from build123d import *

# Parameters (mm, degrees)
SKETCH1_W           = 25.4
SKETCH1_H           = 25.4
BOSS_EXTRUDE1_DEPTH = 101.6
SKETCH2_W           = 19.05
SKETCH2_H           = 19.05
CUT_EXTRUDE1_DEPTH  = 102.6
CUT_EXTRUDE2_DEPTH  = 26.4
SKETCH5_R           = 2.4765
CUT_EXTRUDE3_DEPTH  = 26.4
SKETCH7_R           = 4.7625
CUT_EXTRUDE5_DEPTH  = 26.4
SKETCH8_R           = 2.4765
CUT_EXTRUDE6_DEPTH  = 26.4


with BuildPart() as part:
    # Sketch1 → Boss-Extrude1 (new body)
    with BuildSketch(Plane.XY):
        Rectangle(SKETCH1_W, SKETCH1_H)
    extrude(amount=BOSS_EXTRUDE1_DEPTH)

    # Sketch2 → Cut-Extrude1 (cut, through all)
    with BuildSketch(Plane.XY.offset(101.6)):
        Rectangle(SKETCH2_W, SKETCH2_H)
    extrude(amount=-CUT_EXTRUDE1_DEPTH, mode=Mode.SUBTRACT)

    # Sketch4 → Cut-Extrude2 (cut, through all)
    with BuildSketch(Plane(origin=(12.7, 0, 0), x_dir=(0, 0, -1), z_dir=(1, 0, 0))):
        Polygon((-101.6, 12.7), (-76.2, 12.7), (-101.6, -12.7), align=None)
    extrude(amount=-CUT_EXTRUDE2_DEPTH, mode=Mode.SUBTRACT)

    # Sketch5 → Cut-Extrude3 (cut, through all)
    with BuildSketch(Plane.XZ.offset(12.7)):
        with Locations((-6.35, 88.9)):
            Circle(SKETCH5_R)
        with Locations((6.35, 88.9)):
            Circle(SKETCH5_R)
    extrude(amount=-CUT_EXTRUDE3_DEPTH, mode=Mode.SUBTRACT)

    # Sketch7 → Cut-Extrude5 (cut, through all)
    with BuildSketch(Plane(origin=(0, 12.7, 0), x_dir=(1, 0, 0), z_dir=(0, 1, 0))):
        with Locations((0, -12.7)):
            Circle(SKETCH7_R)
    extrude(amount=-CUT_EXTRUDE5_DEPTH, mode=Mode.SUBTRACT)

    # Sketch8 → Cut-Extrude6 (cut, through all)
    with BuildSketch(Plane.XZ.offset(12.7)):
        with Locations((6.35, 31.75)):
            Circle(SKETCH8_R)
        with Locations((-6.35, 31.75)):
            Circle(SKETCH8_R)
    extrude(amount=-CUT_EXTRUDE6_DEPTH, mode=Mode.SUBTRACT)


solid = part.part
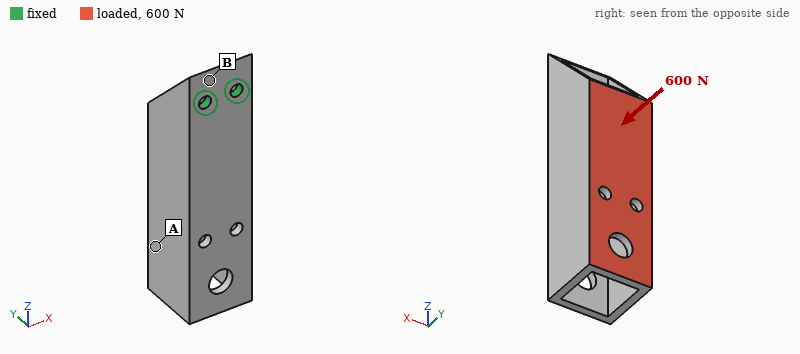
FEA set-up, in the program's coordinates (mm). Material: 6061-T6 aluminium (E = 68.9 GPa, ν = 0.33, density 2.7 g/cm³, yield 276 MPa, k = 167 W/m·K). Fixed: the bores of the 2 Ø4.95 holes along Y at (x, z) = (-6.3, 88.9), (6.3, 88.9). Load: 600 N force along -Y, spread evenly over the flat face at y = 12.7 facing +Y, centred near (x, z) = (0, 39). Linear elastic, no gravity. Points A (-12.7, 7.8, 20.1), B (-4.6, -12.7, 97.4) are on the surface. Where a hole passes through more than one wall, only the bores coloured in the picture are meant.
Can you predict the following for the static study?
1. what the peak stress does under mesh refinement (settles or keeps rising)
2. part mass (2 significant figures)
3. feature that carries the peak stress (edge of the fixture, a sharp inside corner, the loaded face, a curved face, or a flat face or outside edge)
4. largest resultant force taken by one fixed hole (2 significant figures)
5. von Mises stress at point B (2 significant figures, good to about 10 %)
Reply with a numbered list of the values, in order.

1. keeps rising
2. 66 g
3. edge of the fixture
4. 310 N
5. 72 MPa
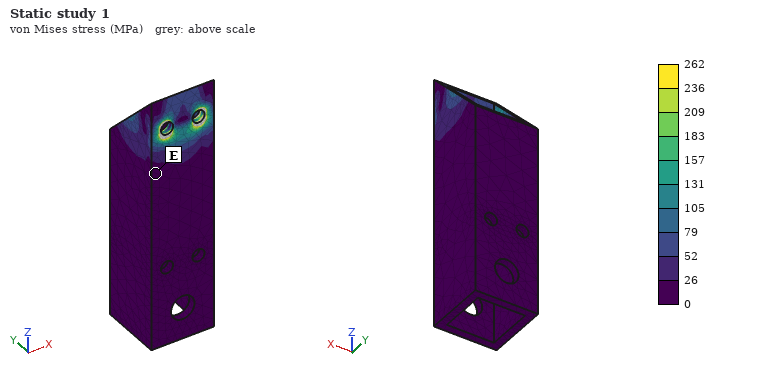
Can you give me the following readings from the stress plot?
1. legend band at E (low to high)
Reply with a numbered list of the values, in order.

1. 0 to 26 MPa
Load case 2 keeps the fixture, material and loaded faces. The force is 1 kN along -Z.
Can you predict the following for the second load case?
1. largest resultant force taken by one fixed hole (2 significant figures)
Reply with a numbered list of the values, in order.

1. 500 N
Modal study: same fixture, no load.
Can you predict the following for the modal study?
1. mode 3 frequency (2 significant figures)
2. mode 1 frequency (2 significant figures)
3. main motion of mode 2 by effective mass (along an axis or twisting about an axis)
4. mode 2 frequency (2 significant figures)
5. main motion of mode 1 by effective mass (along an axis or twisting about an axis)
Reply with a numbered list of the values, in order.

1. 2700 Hz
2. 690 Hz
3. along X
4. 1700 Hz
5. along Y
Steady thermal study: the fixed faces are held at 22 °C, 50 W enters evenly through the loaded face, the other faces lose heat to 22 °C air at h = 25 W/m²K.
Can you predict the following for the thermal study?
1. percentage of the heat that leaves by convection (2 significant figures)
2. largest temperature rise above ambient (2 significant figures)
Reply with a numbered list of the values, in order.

1. 29 %
2. 60 K
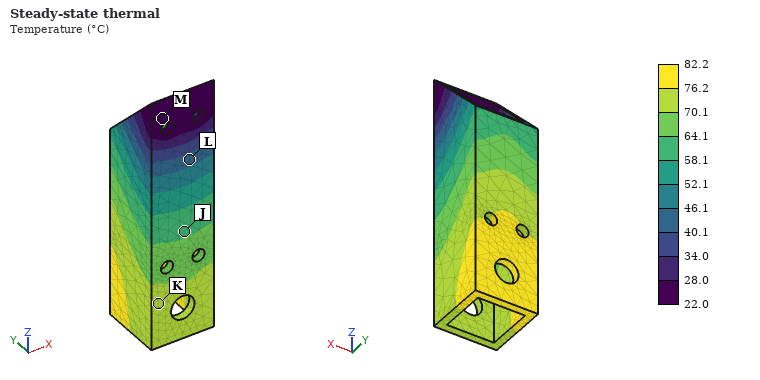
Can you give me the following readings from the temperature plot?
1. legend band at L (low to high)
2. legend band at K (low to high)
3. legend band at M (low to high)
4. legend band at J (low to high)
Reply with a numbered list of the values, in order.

1. 40.1 to 46.1 °C
2. 70.1 to 76.2 °C
3. 22.0 to 28.0 °C
4. 58.1 to 64.1 °C
